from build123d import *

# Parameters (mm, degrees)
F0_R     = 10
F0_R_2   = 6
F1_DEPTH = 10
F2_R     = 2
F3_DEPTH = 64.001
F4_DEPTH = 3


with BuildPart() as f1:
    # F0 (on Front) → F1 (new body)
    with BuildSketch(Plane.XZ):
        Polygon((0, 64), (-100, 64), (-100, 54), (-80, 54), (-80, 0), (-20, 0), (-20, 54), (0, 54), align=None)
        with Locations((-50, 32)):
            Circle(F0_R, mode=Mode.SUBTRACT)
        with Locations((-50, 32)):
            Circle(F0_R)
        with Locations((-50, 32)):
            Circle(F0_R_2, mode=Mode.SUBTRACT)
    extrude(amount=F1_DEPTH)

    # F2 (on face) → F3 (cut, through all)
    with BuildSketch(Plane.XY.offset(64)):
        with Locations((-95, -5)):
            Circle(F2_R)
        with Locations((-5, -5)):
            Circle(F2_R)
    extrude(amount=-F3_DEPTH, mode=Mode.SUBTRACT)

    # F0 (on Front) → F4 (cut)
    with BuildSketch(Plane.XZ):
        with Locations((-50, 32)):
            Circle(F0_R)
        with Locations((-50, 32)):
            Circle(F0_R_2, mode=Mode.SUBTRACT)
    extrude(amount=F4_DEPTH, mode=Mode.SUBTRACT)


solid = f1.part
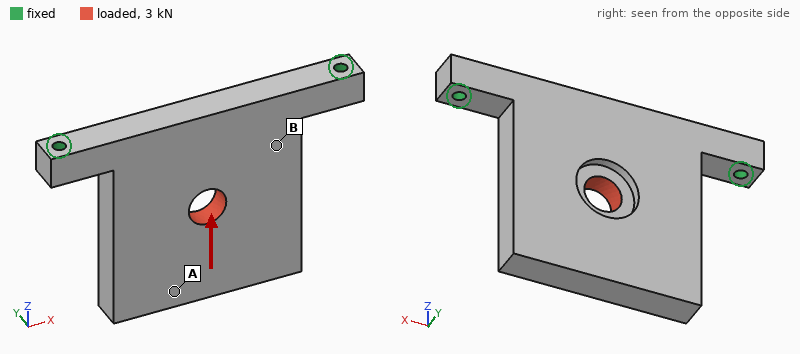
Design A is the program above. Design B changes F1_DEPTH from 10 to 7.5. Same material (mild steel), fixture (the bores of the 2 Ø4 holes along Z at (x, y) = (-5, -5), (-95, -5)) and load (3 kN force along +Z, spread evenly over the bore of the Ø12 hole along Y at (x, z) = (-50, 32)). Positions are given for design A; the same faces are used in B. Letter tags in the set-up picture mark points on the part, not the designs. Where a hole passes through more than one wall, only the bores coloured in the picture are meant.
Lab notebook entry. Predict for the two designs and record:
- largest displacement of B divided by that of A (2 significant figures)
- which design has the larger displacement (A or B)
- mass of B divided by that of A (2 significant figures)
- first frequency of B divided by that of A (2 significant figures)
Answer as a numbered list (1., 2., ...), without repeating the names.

1. 1.8
2. B
3. 0.74
4. 0.84
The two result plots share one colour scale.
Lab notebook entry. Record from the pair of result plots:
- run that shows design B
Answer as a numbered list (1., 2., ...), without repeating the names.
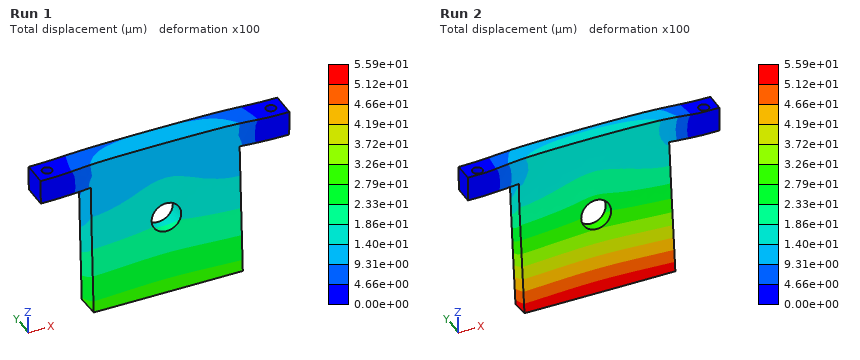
1. Run 2
